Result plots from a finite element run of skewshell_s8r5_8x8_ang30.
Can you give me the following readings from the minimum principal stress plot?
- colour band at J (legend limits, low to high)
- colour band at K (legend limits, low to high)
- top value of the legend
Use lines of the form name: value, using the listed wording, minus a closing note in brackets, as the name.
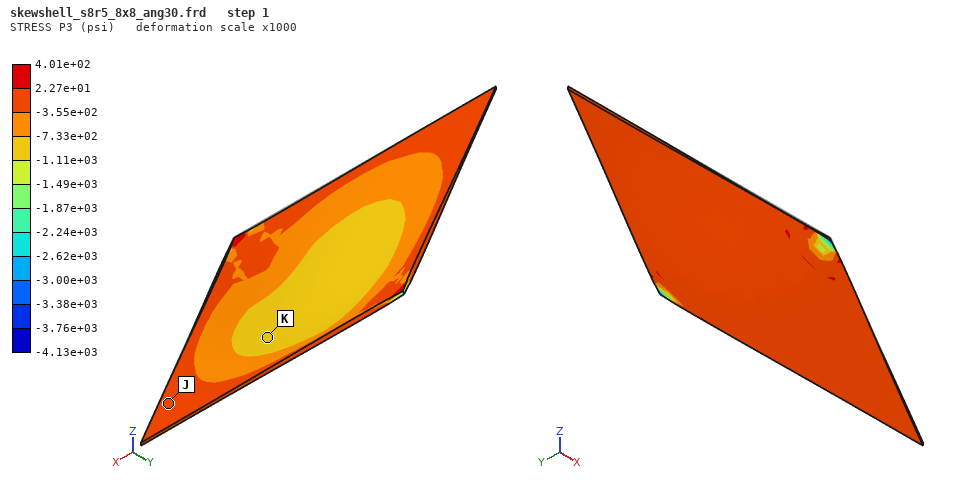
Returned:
colour band at J: -3.55e+02 to 2.27e+01 psi
colour band at K: -1.11e+03 to -7.33e+02 psi
top value of the legend: 4.01e+02 psi
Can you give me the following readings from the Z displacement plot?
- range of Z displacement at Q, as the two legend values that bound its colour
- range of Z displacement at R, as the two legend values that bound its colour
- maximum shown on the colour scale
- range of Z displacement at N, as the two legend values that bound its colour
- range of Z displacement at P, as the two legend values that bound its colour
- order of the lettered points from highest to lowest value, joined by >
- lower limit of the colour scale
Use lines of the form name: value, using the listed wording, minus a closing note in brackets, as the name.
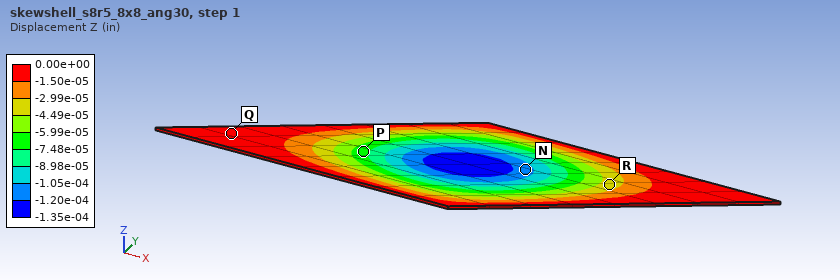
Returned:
range of Z displacement at Q, as the two legend values that bound its colour: -1.50e-05 to 0.00e+00 in
range of Z displacement at R, as the two legend values that bound its colour: -4.49e-05 to -2.99e-05 in
maximum shown on the colour scale: 0.00e+00 in
range of Z displacement at N, as the two legend values that bound its colour: -1.20e-04 to -1.05e-04 in
range of Z displacement at P, as the two legend values that bound its colour: -7.48e-05 to -5.99e-05 in
order of the lettered points from highest to lowest value, joined by >: Q > R > P > N
lower limit of the colour scale: -1.35e-04 in
